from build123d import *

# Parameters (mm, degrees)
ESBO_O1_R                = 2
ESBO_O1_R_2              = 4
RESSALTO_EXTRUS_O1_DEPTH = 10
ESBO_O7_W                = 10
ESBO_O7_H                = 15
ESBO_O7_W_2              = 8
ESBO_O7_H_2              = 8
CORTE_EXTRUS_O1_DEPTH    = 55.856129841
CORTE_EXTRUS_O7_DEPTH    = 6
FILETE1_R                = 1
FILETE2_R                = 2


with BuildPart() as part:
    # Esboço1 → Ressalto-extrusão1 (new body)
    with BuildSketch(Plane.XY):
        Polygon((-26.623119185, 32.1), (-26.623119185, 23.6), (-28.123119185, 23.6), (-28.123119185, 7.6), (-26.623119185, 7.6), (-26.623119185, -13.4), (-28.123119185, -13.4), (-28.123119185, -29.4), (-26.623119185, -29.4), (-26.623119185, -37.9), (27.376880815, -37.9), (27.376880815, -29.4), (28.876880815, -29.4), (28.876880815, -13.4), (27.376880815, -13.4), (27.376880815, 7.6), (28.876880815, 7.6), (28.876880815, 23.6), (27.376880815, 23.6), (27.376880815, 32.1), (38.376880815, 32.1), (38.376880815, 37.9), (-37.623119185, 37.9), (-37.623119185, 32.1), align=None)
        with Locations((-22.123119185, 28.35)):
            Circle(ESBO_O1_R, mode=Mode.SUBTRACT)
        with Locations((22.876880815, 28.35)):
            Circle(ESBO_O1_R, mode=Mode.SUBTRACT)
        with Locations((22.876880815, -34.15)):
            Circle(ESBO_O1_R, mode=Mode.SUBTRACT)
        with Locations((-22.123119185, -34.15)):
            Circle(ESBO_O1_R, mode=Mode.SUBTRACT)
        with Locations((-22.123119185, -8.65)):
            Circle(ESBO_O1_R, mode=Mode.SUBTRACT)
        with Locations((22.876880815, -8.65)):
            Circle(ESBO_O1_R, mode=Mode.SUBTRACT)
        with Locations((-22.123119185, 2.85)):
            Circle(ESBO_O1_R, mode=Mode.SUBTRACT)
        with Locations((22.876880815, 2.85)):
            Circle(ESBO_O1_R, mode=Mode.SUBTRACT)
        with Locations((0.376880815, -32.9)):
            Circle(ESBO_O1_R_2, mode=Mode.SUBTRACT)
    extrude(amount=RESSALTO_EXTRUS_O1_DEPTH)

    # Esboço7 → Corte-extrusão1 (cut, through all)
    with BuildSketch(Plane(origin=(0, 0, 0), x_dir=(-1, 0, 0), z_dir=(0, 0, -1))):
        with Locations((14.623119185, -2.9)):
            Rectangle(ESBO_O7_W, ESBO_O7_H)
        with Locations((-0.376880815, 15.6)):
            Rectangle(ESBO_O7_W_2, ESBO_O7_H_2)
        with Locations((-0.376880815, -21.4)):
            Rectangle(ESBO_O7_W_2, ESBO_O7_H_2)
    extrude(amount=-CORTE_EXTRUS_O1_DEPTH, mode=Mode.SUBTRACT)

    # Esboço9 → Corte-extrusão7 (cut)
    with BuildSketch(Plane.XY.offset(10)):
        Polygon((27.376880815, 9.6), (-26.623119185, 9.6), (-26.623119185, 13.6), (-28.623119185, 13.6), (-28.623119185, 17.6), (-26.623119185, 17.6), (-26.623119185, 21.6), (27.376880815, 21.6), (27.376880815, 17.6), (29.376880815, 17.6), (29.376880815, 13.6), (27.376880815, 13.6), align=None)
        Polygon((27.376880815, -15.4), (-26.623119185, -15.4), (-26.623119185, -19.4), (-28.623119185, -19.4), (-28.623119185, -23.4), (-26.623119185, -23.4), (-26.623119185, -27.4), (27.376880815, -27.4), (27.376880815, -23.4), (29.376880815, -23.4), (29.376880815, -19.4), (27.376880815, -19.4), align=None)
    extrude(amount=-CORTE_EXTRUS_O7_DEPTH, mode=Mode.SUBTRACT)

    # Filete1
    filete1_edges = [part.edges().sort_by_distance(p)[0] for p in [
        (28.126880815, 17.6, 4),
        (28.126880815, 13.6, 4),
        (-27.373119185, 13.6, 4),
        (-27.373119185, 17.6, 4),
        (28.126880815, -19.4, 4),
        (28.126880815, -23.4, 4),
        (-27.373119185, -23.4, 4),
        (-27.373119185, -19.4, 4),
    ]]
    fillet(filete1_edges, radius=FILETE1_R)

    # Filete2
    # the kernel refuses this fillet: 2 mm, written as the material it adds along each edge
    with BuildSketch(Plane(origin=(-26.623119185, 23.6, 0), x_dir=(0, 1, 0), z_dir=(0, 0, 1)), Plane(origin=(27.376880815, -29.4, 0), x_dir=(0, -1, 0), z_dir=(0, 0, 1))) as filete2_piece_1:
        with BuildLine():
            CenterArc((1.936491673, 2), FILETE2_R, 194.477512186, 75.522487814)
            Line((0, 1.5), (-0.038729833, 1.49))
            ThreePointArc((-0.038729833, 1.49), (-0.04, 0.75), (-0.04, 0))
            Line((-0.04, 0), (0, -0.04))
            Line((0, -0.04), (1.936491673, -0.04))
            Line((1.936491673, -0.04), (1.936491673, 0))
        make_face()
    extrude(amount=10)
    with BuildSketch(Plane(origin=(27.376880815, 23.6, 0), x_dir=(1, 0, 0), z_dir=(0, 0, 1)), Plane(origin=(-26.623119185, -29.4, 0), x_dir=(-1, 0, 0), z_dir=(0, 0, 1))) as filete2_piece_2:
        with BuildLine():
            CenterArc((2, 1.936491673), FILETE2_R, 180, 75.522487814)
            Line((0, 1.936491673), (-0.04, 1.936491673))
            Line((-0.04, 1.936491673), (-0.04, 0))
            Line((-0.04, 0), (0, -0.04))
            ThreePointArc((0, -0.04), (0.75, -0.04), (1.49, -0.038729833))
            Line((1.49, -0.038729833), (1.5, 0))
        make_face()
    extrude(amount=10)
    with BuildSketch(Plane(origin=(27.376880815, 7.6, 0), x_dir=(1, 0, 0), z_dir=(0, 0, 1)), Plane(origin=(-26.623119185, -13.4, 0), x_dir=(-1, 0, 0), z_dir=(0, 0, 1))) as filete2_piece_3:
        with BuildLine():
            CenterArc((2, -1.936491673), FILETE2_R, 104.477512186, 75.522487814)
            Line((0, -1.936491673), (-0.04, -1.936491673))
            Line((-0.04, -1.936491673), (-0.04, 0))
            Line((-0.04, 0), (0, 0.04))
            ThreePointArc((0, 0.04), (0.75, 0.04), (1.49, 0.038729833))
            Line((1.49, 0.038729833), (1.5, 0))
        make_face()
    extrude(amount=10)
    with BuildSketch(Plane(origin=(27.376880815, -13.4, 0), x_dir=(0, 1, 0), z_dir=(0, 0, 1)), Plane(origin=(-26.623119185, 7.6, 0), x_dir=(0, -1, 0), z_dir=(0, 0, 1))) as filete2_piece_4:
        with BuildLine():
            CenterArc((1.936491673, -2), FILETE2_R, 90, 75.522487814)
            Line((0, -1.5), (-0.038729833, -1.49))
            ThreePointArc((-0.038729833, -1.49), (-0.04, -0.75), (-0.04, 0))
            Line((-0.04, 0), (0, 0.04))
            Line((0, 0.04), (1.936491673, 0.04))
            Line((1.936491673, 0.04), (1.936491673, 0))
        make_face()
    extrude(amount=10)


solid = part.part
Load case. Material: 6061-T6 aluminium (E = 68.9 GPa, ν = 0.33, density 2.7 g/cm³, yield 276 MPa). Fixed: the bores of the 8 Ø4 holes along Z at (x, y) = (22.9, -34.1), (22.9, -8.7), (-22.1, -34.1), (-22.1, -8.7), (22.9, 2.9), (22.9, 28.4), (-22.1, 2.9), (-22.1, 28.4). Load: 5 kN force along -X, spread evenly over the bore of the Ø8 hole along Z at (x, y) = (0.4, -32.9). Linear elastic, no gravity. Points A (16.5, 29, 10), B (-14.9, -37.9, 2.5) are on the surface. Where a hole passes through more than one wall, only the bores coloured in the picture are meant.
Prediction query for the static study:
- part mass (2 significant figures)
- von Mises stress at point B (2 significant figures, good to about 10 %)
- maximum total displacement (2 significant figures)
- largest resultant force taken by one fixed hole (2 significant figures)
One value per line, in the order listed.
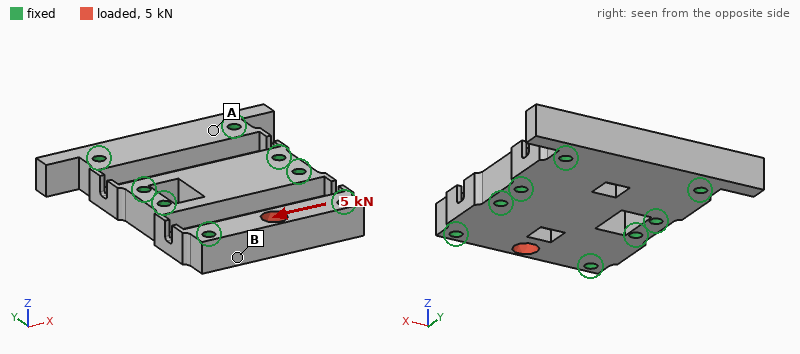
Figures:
86 g
26 MPa
8.3 µm
2.2 kN
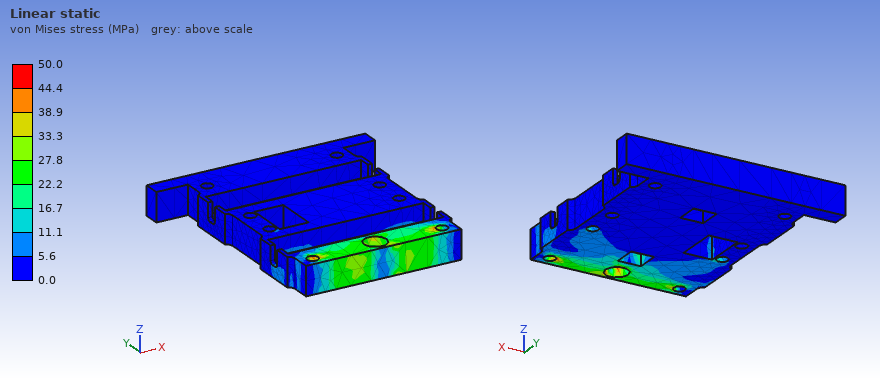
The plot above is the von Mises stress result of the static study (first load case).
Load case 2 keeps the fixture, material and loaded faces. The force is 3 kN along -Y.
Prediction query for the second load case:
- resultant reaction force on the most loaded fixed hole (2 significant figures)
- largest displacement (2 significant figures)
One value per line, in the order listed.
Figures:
900 N
24 µm
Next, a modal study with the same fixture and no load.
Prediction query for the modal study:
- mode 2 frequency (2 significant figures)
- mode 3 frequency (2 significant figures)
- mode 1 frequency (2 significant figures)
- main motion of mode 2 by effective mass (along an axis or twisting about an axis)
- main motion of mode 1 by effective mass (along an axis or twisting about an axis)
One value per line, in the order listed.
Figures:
19 kHz
20 kHz
17 kHz
twisting about X
along Z
